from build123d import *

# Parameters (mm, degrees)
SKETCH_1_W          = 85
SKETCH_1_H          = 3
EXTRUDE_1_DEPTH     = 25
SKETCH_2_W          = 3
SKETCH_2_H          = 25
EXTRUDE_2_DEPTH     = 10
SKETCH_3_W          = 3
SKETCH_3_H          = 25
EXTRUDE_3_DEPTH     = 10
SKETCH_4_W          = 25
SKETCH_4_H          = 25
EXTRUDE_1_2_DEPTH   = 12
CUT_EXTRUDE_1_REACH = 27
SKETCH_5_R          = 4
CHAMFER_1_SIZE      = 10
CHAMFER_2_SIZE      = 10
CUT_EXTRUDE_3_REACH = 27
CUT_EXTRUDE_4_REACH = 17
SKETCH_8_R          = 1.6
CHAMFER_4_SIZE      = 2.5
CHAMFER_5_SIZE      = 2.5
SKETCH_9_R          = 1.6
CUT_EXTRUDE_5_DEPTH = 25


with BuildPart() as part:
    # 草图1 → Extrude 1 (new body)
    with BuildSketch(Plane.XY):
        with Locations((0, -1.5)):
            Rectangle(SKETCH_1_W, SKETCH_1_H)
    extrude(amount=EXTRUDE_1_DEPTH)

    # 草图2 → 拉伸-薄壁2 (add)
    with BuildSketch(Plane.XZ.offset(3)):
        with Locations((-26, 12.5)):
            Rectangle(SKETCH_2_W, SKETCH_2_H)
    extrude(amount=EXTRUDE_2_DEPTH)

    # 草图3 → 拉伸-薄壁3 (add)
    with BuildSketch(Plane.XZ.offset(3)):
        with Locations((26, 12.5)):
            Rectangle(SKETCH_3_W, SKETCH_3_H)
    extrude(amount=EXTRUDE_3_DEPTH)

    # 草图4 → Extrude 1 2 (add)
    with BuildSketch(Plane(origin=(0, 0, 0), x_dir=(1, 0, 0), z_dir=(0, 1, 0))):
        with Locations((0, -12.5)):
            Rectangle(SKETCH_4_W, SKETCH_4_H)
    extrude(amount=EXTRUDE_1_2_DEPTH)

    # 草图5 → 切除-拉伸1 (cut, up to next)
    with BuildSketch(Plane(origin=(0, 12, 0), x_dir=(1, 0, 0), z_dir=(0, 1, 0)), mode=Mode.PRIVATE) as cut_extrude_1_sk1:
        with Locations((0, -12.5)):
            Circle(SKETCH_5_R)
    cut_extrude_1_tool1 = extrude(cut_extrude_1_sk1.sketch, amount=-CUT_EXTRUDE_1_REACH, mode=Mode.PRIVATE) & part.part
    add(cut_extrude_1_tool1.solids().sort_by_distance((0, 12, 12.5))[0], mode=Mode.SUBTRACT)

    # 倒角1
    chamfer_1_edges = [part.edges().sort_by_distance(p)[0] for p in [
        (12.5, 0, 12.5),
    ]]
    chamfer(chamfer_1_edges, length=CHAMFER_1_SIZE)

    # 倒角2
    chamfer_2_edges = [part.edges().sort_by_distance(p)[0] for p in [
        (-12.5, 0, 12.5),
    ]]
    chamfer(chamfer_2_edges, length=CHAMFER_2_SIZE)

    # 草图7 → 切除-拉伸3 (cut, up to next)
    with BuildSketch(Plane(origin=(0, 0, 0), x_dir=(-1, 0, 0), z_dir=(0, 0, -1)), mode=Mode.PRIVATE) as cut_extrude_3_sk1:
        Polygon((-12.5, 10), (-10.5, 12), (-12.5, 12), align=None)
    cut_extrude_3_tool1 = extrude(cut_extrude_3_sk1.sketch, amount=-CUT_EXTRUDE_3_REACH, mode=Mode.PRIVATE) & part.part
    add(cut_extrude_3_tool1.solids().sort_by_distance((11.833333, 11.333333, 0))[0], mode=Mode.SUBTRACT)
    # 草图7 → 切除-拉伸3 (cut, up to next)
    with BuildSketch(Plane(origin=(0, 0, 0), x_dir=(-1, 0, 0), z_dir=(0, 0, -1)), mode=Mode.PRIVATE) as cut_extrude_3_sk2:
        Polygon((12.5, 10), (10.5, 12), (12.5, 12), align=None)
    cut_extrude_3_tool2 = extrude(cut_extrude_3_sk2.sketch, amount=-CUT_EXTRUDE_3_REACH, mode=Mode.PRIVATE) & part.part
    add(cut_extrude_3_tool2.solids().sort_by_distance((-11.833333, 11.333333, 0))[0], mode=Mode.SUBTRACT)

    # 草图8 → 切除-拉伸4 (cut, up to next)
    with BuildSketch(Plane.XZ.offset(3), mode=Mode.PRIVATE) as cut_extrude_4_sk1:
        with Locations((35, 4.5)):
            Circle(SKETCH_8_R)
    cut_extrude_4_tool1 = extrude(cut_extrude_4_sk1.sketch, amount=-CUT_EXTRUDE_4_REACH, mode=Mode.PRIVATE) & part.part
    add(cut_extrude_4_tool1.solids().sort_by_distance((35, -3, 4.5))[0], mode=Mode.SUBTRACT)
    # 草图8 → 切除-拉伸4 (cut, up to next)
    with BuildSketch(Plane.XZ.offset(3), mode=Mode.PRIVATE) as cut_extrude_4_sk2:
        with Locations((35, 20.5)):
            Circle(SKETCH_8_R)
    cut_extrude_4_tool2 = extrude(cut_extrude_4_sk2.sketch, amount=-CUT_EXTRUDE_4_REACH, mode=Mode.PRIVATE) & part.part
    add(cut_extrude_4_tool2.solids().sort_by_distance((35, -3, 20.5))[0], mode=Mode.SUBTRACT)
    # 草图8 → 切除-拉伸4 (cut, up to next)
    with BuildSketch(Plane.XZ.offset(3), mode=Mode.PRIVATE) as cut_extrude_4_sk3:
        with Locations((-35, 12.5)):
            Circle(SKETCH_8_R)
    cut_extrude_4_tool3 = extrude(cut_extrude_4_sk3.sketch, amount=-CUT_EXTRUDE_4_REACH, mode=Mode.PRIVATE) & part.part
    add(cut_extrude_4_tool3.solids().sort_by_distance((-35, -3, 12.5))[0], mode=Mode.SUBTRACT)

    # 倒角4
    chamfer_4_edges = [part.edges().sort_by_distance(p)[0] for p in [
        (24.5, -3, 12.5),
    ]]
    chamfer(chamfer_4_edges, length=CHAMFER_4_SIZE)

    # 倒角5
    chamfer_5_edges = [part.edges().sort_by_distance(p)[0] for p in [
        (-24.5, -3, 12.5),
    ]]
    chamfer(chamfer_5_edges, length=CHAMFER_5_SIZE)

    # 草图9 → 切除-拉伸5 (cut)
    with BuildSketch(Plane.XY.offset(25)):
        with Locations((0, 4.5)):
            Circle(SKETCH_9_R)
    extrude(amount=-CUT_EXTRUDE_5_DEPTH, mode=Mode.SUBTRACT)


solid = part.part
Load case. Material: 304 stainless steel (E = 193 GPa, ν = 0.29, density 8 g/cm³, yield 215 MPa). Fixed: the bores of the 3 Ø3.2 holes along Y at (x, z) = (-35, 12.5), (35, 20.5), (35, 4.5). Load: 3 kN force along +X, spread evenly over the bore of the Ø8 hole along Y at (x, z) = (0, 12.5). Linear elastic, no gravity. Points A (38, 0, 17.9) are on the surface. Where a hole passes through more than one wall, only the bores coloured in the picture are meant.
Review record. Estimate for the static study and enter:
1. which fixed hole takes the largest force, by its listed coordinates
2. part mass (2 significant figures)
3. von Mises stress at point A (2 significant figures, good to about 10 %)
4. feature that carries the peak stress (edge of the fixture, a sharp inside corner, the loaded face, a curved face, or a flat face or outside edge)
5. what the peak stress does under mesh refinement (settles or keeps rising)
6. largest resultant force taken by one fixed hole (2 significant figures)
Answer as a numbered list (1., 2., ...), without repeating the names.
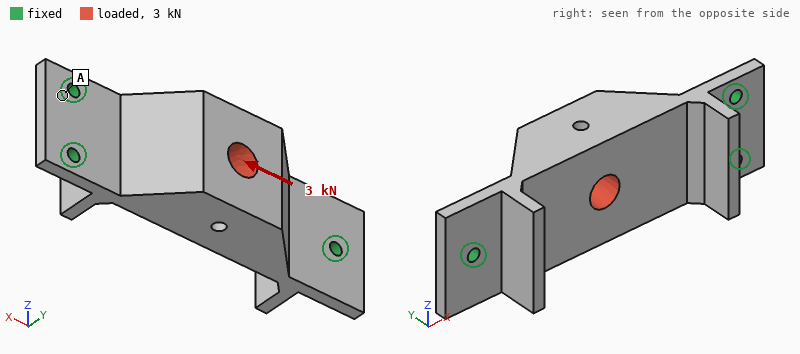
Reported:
1. (-35, 12.5)
2. 140 g
3. 8.5 MPa
4. edge of the fixture
5. keeps rising
6. 1.4 kN
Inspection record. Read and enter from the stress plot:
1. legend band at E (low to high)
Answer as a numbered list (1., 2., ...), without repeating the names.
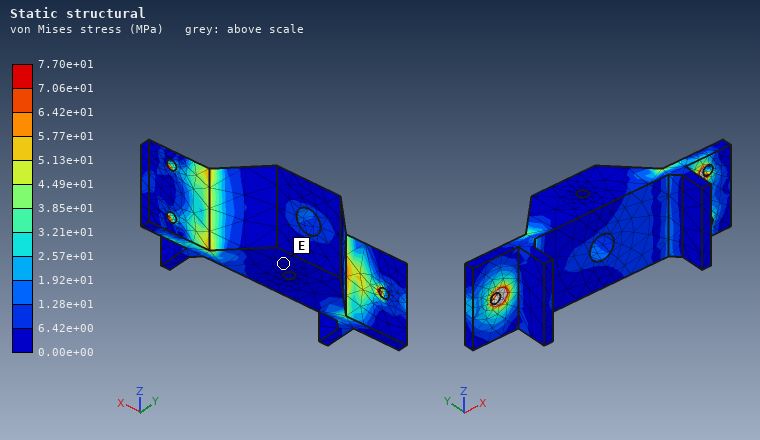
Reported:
1. 0.00e+00 to 6.42e+00 MPa
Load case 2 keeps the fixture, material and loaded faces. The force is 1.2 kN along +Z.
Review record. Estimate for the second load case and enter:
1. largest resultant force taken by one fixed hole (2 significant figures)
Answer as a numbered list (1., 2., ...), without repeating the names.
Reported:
1. 780 N
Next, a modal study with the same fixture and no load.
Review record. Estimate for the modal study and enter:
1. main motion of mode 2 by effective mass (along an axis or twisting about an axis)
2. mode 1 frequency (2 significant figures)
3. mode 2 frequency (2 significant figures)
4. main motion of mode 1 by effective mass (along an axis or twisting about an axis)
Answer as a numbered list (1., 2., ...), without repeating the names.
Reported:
1. along Y
2. 3600 Hz
3. 3800 Hz
4. along Z
